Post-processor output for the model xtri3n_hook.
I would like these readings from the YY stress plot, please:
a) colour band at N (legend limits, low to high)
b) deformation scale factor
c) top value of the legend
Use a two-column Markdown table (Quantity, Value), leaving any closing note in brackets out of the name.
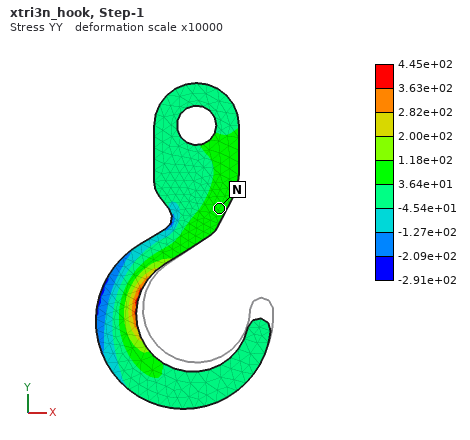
| Quantity | Value |
|---|---|
| colour band at N | 3.64e+01 to 1.18e+02 |
| deformation scale factor | 10000 |
| top value of the legend | 4.45e+02 |
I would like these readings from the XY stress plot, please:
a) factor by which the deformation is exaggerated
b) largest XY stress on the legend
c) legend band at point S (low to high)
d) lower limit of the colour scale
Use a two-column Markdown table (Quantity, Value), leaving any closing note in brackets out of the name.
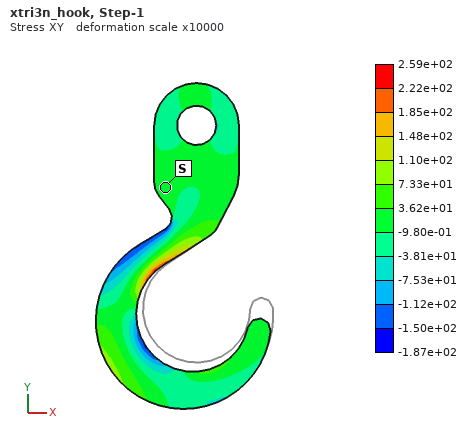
| Quantity | Value |
|---|---|
| factor by which the deformation is exaggerated | 10000 |
| largest XY stress on the legend | 2.59e+02 |
| legend band at point S | -9.80e-01 to 3.62e+01 |
| lower limit of the colour scale | -1.87e+02 |
